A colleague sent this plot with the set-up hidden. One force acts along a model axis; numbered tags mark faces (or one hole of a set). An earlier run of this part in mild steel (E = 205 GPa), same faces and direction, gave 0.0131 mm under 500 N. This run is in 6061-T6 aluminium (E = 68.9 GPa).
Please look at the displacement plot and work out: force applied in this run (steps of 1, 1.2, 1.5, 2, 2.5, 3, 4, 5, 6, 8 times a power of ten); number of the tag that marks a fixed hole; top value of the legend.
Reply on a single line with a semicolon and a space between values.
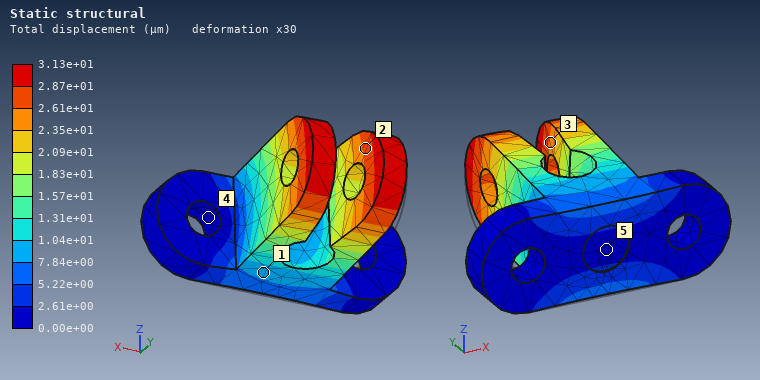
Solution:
400 N; 4; 3.13e+01 µm
